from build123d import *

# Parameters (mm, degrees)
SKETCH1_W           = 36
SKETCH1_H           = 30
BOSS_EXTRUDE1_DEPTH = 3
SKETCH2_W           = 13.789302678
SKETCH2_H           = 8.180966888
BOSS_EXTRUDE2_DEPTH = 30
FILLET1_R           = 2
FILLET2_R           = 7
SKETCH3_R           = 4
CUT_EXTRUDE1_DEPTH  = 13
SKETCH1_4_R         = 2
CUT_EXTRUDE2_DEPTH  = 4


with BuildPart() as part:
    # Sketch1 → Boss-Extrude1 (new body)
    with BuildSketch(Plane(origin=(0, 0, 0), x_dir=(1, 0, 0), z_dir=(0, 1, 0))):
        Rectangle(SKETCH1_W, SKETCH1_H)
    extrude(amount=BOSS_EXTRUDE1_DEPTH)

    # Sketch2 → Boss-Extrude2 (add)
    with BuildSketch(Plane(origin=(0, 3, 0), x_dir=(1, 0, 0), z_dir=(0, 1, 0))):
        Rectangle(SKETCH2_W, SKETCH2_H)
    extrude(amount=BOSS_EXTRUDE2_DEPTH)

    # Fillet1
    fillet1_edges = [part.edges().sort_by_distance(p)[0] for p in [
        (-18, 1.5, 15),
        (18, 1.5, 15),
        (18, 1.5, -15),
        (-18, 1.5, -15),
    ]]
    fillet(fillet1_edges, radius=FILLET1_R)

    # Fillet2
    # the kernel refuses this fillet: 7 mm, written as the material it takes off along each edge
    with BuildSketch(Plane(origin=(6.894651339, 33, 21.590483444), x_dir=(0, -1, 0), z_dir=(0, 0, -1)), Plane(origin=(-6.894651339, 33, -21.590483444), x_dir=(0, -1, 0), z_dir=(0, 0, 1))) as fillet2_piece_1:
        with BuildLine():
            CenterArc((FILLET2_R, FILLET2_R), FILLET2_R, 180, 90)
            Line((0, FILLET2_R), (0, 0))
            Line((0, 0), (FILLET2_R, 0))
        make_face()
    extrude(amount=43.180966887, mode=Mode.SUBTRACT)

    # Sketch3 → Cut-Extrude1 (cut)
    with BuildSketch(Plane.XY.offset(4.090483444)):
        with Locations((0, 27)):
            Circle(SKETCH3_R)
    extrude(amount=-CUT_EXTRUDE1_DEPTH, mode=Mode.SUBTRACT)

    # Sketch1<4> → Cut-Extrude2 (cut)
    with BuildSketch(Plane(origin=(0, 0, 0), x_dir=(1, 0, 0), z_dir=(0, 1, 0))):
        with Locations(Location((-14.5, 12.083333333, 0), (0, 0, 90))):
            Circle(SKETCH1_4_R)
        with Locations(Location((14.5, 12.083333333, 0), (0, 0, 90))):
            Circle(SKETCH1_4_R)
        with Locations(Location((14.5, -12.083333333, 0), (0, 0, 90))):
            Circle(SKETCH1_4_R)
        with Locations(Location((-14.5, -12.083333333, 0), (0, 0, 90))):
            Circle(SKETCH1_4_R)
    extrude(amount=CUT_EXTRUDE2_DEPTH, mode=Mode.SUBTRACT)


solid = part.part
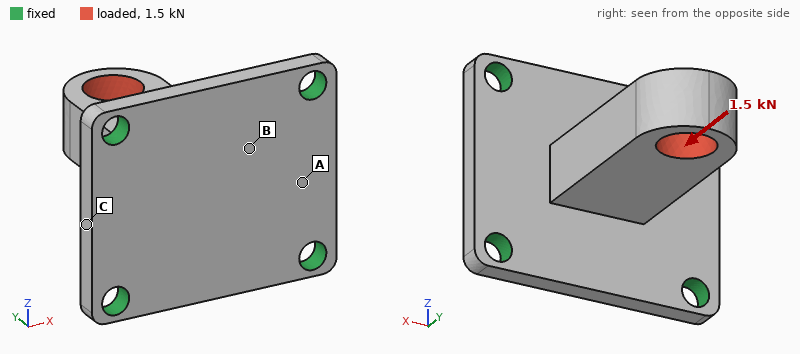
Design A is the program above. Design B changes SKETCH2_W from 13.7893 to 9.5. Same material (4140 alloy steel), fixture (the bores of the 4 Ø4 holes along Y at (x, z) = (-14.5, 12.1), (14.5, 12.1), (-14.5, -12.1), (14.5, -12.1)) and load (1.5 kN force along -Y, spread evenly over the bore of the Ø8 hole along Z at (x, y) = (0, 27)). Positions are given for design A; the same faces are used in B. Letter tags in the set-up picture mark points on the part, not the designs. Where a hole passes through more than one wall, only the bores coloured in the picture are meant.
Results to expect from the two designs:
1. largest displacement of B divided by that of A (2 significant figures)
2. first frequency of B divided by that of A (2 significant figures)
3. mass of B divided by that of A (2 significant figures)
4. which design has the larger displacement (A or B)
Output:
1.5
1.1
0.84
B
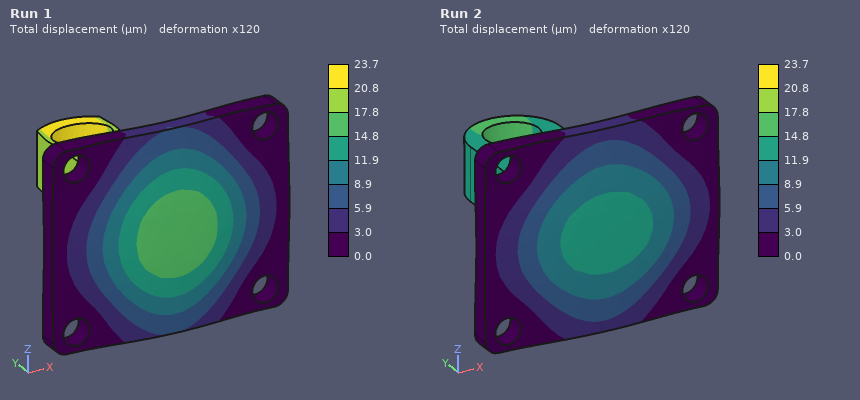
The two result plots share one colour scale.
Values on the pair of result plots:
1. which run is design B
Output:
Run 1
